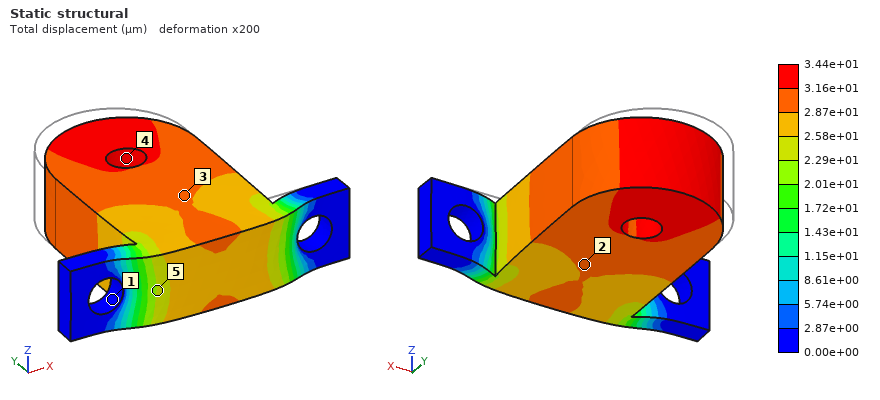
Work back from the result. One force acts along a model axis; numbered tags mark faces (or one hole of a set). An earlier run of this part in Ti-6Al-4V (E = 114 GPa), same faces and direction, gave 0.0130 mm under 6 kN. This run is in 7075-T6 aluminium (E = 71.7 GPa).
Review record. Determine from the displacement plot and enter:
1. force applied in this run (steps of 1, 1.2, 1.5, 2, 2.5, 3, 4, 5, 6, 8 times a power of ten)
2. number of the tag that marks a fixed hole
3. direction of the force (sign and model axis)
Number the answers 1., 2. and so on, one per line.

1. 10 kN
2. 1
3. -Y
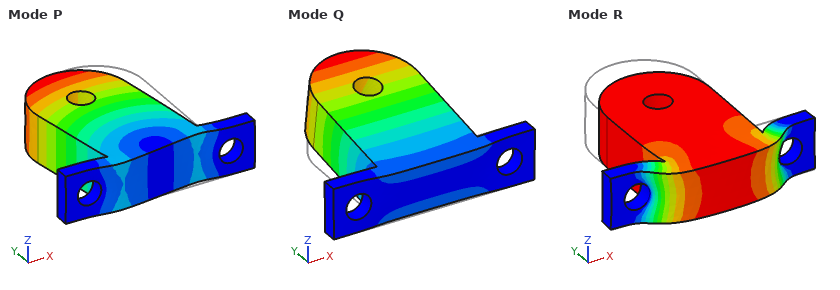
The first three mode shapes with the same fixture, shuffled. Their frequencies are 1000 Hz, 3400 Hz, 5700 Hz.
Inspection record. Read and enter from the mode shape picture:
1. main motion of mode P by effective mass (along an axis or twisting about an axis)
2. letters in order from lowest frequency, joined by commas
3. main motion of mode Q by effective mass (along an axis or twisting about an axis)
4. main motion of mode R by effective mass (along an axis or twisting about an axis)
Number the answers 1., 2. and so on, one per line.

1. along X
2. Q, P, R
3. along Z
4. along Y
